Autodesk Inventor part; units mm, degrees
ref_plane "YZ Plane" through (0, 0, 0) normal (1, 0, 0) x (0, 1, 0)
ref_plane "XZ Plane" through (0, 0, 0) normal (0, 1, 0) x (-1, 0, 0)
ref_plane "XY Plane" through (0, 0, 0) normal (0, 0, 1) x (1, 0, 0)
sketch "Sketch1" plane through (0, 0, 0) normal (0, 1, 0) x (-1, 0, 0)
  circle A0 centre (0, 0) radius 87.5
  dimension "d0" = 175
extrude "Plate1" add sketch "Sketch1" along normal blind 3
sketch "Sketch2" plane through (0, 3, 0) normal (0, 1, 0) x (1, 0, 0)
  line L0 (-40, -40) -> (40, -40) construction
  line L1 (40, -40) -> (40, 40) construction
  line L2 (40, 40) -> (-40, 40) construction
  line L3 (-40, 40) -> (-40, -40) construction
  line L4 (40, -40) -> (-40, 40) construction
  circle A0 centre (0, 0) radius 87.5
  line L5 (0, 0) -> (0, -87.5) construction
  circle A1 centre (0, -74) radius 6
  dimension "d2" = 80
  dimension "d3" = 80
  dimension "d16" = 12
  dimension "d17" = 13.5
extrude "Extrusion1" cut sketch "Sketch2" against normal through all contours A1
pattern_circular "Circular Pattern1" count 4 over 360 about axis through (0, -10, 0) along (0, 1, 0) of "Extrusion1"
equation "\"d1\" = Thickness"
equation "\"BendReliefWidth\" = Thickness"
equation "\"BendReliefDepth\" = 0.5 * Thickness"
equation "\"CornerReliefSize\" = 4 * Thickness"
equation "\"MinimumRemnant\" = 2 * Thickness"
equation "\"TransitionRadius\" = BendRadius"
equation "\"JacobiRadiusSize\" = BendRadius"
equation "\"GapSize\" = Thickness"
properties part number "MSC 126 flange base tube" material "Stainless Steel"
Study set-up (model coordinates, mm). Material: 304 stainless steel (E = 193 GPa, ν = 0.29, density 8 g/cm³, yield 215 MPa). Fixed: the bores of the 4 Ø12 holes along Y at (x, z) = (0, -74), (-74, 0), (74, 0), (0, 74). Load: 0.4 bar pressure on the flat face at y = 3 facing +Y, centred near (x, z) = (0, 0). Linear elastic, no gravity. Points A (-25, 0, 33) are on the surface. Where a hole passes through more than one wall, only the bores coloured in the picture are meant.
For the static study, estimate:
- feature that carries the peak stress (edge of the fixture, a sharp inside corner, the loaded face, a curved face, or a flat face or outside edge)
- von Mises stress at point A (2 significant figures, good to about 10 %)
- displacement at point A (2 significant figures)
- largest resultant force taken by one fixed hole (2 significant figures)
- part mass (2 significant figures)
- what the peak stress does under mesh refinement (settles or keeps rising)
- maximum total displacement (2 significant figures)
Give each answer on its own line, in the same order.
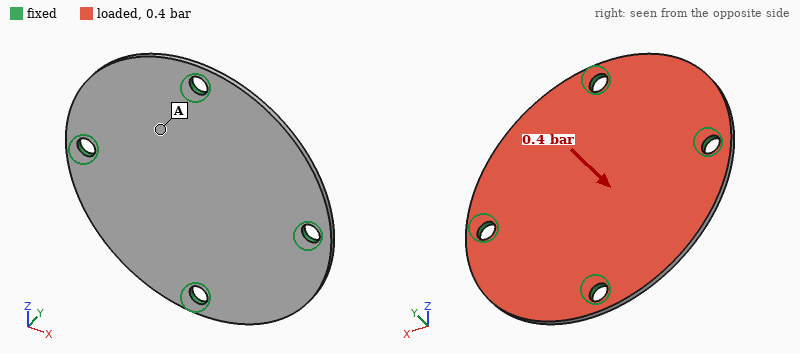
edge of the fixture
13 MPa
34 µm
240 N
570 g
keeps rising
49 µm
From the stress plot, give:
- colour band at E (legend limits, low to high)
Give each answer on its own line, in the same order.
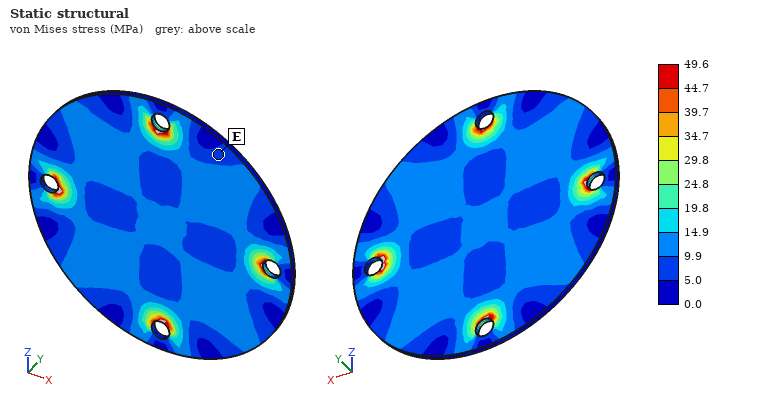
5.0 to 9.9 MPa
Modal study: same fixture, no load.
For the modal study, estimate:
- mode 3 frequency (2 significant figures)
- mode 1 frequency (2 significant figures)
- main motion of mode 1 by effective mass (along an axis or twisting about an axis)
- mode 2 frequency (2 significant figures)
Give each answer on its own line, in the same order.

1300 Hz
1100 Hz
along Y
1300 Hz
